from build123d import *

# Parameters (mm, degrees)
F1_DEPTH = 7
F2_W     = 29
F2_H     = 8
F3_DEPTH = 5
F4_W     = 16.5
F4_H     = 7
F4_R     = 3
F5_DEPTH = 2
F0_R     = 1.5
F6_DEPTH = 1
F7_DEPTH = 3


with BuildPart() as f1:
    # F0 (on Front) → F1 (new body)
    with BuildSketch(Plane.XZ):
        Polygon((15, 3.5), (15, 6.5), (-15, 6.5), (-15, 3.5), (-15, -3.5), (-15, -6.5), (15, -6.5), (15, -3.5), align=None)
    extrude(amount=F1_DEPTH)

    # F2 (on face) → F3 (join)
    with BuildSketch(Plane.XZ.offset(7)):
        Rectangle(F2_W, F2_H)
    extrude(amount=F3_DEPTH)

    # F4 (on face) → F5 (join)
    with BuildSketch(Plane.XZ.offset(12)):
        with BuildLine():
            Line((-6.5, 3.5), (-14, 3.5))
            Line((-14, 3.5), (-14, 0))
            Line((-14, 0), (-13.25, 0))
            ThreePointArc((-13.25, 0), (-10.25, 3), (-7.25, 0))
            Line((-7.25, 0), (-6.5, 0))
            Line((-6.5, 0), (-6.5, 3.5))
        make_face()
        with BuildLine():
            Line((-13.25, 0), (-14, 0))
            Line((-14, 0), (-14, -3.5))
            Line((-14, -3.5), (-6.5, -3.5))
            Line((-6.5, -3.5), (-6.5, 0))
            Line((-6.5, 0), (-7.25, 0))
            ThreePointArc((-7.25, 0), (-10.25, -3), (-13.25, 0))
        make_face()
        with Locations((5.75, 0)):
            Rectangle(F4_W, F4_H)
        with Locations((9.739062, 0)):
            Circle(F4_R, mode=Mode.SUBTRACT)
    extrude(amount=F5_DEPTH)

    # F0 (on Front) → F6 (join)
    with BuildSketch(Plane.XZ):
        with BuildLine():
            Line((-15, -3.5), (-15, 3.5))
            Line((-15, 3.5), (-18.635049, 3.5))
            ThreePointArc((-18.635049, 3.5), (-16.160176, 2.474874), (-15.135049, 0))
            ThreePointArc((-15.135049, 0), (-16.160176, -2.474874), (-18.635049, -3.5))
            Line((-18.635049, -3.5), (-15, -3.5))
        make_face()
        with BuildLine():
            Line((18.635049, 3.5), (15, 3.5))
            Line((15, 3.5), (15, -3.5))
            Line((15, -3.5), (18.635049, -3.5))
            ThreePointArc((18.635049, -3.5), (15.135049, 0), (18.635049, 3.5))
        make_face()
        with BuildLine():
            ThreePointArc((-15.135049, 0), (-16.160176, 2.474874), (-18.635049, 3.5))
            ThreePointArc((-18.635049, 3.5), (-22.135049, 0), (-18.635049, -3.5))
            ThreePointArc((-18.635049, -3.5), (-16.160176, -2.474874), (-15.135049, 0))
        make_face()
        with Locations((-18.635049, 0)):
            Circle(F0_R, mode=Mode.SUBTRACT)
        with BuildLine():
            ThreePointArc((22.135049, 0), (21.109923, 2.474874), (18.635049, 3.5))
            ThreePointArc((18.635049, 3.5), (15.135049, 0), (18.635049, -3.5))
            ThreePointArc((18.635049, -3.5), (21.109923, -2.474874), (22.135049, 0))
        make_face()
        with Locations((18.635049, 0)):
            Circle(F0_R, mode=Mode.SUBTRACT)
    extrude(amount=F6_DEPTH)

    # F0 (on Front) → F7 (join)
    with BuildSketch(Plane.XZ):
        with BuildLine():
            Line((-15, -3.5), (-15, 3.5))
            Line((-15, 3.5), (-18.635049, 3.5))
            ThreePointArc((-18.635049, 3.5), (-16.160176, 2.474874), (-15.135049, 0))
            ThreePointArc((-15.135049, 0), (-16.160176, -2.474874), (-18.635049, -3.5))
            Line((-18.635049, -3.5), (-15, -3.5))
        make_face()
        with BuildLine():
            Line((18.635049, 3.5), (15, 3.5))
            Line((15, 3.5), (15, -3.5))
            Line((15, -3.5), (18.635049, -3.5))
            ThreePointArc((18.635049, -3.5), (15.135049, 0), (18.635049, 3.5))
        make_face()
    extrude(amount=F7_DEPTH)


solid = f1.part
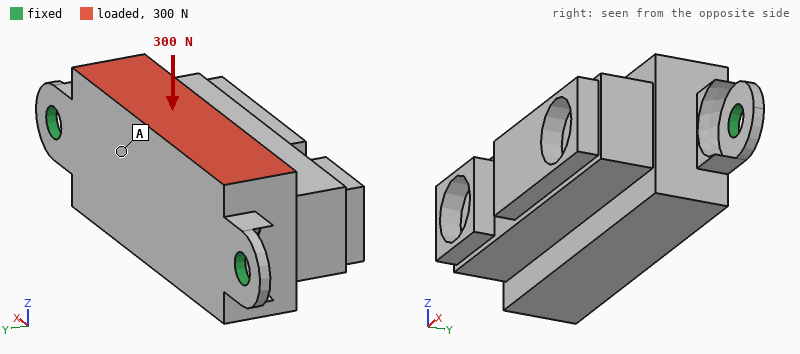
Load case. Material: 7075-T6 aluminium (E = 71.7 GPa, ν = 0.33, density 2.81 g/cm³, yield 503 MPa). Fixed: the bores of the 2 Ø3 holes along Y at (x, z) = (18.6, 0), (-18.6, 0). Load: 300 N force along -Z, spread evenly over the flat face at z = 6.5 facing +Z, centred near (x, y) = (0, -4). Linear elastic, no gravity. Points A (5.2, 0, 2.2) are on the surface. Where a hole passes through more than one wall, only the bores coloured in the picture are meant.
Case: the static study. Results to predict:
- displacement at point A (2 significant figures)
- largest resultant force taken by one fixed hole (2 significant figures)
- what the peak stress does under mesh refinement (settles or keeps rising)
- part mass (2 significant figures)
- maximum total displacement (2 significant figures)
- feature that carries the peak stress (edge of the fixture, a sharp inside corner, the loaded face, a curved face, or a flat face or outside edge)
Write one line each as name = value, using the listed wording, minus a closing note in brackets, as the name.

displacement at point A = 11 µm
largest resultant force taken by one fixed hole = 150 N
what the peak stress does under mesh refinement = keeps rising
part mass = 12 g
maximum total displacement = 74 µm
feature that carries the peak stress = edge of the fixture
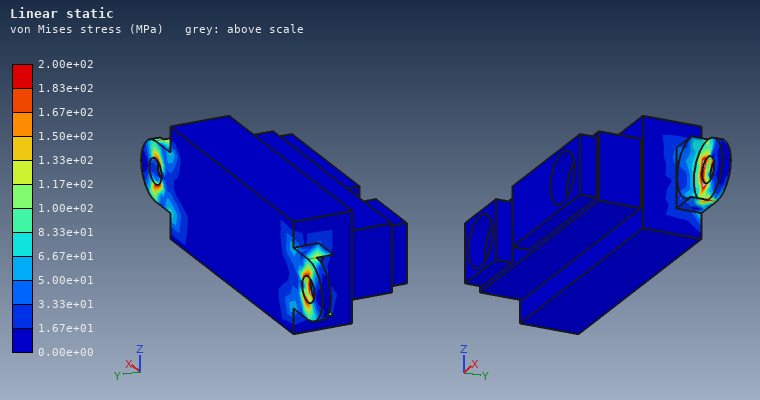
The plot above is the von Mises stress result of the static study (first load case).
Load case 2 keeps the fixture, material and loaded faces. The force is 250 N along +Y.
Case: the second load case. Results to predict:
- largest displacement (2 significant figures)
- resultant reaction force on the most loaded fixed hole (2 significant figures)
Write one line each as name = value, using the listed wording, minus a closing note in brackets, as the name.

largest displacement = 0.13 mm
resultant reaction force on the most loaded fixed hole = 160 N
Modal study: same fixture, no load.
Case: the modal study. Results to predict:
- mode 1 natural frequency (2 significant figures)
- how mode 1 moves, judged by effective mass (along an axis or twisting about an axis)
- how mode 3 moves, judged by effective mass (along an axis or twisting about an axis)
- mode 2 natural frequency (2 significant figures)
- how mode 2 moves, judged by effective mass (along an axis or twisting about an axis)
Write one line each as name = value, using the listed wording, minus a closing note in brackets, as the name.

mode 1 natural frequency = 2700 Hz
how mode 1 moves, judged by effective mass = along Z
how mode 3 moves, judged by effective mass = along X
mode 2 natural frequency = 9300 Hz
how mode 2 moves, judged by effective mass = along Y
